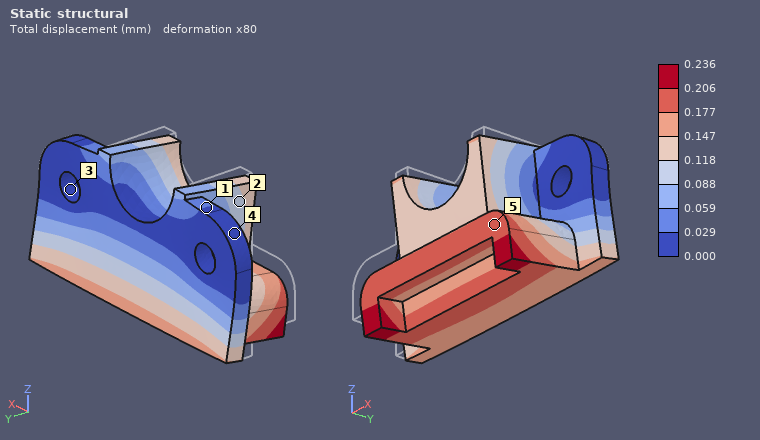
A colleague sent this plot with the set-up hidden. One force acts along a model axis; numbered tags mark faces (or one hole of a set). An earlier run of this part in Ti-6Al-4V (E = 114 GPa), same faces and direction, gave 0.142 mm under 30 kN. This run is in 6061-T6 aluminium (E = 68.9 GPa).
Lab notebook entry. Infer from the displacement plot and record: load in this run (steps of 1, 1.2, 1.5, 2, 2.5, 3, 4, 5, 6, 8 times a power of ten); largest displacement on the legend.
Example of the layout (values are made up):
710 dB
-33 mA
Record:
30 kN
0.236 mm
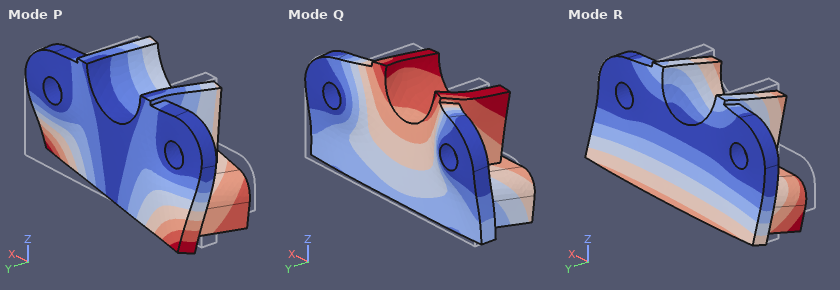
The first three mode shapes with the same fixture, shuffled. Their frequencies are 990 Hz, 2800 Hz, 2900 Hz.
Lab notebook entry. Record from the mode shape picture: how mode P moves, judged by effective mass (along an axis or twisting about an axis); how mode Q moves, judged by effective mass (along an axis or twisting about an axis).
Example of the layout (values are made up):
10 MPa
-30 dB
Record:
along X
along Y
